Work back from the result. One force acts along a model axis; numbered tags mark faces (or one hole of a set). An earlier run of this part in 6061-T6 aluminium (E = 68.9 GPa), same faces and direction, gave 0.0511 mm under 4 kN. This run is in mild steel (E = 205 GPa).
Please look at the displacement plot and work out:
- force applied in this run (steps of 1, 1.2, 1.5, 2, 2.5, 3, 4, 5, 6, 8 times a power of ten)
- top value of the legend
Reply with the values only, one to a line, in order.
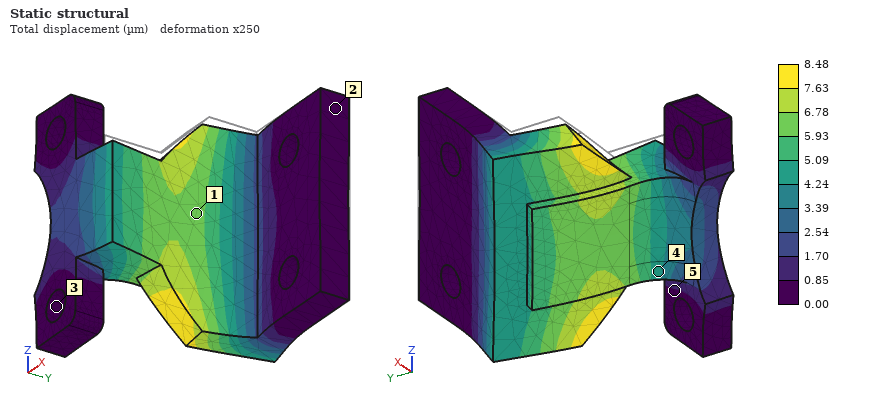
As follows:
2 kN
8.48 µm
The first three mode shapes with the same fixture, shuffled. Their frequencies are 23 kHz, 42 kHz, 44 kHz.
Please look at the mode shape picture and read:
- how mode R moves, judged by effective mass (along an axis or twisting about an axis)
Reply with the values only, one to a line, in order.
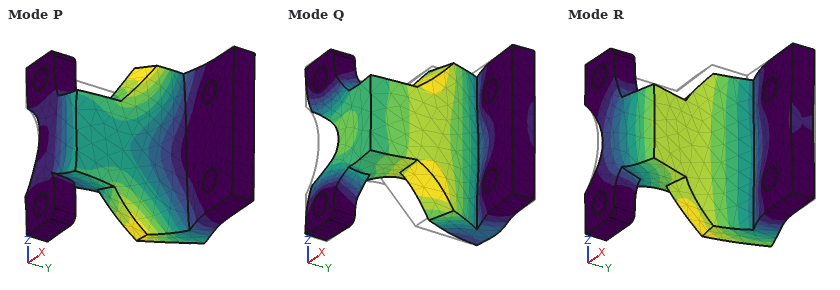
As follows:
along Y
